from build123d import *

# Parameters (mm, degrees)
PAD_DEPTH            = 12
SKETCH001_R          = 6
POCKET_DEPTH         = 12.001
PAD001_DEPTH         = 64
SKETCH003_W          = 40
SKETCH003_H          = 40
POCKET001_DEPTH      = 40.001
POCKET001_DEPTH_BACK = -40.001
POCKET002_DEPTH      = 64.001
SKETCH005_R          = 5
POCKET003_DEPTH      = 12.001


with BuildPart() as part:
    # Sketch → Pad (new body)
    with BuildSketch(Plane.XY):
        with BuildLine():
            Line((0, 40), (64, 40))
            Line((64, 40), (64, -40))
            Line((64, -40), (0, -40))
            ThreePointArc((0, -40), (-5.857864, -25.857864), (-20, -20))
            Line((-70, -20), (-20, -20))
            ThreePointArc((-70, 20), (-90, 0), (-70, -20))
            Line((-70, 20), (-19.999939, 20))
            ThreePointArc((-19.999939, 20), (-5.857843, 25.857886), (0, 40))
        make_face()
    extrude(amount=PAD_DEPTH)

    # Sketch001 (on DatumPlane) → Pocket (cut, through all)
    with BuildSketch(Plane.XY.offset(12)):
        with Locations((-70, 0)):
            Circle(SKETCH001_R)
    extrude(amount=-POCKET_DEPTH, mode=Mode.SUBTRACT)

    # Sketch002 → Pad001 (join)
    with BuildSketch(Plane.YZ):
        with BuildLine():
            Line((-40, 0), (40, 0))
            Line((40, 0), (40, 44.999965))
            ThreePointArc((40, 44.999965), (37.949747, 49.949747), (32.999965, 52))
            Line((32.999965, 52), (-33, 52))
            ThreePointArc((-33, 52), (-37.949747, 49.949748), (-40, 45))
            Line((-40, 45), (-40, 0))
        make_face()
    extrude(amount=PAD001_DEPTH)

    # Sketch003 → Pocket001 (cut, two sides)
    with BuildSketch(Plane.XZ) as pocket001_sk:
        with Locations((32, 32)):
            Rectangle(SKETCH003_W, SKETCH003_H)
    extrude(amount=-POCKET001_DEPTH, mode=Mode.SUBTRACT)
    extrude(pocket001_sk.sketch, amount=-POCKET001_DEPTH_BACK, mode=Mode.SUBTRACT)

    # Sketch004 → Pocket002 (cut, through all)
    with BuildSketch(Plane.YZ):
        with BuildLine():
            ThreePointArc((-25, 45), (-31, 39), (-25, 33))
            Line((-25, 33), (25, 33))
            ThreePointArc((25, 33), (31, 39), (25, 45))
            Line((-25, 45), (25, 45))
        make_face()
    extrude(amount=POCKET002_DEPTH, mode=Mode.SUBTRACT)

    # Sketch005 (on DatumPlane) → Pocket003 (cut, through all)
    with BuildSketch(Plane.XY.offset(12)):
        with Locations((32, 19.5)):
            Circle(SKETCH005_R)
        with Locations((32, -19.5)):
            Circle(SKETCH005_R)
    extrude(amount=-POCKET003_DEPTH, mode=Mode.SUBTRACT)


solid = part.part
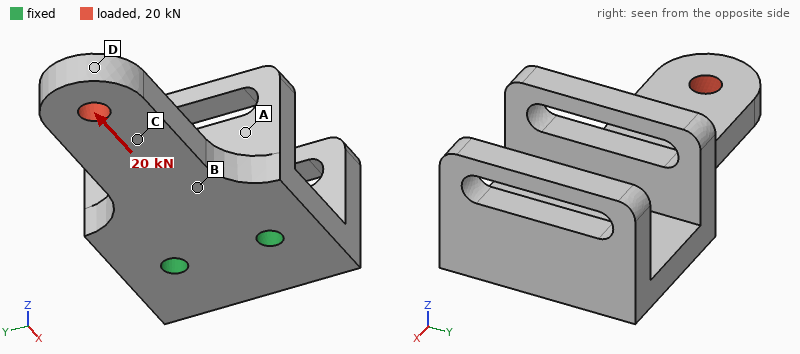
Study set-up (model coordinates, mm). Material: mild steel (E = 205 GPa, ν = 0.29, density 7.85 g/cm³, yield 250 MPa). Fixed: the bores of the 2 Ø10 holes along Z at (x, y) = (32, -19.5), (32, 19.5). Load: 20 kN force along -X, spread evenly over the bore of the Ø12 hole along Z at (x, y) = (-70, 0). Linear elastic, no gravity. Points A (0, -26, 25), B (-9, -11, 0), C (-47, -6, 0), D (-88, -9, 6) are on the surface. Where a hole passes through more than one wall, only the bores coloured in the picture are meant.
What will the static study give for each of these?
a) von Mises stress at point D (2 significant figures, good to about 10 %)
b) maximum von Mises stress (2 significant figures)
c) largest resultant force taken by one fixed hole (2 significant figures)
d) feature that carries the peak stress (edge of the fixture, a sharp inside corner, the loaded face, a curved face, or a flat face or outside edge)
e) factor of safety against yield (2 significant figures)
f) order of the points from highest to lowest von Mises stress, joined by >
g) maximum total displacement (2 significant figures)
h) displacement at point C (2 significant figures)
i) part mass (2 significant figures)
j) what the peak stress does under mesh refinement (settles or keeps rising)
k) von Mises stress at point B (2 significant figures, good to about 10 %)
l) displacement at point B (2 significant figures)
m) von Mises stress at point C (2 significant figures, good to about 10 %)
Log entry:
25 MPa
120 MPa
10 kN
the loaded face
2.2
C > B > D > A
24 µm
15 µm
1.3 kg
settles
34 MPa
6.8 µm
44 MPa
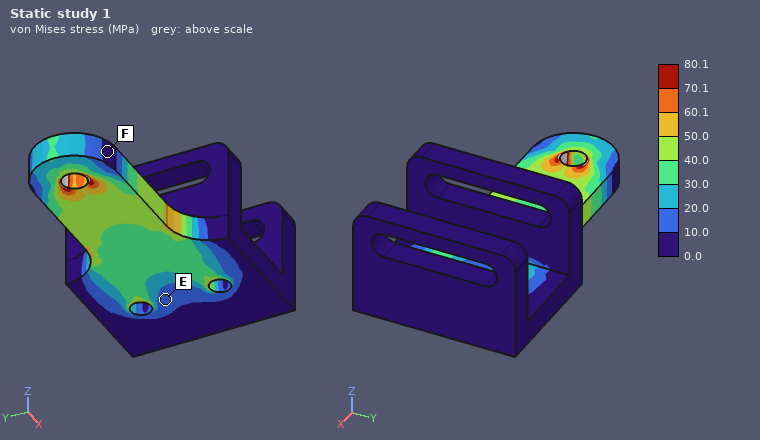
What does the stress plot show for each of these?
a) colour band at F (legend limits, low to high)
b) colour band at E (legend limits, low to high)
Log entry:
0.0 to 10.0 MPa
10.0 to 20.0 MPa
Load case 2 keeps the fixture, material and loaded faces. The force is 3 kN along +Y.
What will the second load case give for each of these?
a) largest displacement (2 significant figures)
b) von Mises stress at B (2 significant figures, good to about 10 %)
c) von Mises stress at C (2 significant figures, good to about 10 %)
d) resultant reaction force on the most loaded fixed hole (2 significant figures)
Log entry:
53 µm
17 MPa
16 MPa
7.0 kN
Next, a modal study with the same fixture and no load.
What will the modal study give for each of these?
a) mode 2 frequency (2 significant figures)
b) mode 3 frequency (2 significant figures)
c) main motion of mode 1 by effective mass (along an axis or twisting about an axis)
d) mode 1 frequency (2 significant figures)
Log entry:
2800 Hz
3100 Hz
along Z
940 Hz
